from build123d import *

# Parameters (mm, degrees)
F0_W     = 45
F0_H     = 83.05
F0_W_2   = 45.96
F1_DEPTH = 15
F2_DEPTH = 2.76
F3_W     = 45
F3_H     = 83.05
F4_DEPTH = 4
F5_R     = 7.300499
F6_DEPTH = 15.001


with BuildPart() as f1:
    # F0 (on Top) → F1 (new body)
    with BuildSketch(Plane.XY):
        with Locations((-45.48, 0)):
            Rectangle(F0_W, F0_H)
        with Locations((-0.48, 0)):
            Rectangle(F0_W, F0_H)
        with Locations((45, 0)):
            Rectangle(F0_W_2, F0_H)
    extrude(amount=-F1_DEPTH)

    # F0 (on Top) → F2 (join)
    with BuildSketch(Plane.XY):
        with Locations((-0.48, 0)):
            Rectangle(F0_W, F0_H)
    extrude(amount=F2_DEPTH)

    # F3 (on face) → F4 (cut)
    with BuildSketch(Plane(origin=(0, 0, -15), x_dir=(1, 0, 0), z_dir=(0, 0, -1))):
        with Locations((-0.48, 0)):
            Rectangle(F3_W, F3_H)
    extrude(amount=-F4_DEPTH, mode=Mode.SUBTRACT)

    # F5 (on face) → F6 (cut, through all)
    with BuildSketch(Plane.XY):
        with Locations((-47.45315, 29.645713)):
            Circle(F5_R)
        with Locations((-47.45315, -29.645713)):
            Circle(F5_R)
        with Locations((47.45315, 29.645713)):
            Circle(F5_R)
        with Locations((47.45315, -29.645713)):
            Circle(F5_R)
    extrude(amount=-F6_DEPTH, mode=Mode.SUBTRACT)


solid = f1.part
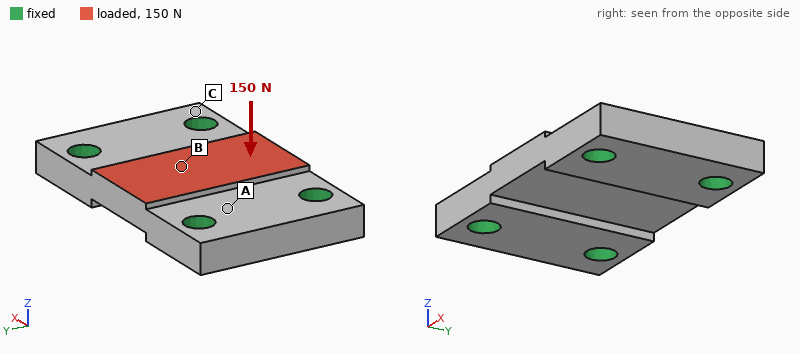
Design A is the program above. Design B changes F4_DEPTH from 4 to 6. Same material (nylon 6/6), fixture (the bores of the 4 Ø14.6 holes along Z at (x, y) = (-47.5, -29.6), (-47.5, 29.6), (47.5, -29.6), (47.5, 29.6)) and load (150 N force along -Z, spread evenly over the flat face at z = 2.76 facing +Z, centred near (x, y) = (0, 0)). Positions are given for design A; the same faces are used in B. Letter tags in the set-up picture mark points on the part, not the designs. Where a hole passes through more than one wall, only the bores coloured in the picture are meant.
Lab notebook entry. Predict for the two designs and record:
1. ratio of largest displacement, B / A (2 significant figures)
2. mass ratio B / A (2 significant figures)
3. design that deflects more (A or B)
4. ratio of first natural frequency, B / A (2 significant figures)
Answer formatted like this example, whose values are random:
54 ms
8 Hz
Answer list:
1.1
0.95
B
1.0
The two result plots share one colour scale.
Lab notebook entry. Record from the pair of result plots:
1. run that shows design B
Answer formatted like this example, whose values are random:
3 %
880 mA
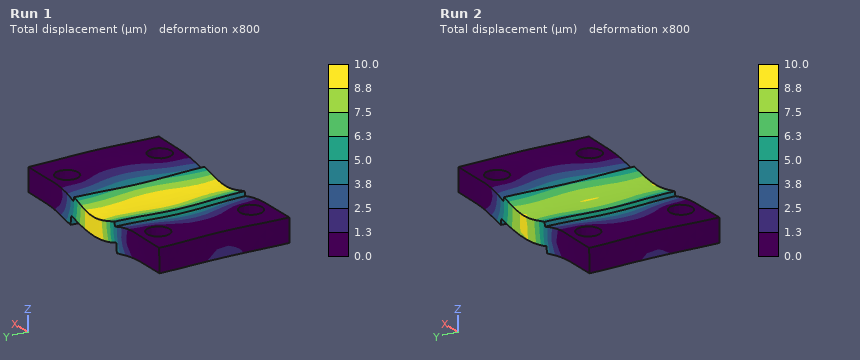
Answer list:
Run 1
